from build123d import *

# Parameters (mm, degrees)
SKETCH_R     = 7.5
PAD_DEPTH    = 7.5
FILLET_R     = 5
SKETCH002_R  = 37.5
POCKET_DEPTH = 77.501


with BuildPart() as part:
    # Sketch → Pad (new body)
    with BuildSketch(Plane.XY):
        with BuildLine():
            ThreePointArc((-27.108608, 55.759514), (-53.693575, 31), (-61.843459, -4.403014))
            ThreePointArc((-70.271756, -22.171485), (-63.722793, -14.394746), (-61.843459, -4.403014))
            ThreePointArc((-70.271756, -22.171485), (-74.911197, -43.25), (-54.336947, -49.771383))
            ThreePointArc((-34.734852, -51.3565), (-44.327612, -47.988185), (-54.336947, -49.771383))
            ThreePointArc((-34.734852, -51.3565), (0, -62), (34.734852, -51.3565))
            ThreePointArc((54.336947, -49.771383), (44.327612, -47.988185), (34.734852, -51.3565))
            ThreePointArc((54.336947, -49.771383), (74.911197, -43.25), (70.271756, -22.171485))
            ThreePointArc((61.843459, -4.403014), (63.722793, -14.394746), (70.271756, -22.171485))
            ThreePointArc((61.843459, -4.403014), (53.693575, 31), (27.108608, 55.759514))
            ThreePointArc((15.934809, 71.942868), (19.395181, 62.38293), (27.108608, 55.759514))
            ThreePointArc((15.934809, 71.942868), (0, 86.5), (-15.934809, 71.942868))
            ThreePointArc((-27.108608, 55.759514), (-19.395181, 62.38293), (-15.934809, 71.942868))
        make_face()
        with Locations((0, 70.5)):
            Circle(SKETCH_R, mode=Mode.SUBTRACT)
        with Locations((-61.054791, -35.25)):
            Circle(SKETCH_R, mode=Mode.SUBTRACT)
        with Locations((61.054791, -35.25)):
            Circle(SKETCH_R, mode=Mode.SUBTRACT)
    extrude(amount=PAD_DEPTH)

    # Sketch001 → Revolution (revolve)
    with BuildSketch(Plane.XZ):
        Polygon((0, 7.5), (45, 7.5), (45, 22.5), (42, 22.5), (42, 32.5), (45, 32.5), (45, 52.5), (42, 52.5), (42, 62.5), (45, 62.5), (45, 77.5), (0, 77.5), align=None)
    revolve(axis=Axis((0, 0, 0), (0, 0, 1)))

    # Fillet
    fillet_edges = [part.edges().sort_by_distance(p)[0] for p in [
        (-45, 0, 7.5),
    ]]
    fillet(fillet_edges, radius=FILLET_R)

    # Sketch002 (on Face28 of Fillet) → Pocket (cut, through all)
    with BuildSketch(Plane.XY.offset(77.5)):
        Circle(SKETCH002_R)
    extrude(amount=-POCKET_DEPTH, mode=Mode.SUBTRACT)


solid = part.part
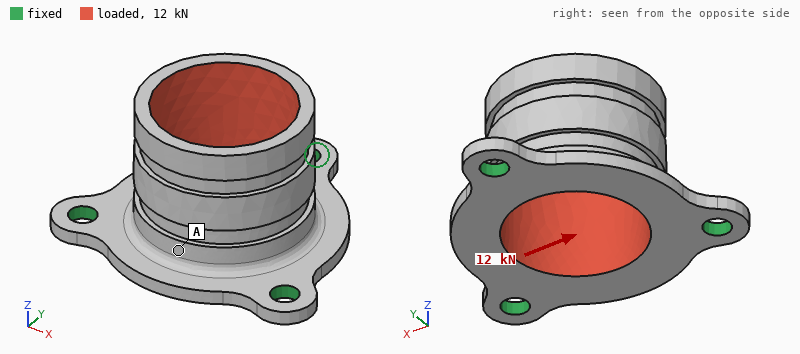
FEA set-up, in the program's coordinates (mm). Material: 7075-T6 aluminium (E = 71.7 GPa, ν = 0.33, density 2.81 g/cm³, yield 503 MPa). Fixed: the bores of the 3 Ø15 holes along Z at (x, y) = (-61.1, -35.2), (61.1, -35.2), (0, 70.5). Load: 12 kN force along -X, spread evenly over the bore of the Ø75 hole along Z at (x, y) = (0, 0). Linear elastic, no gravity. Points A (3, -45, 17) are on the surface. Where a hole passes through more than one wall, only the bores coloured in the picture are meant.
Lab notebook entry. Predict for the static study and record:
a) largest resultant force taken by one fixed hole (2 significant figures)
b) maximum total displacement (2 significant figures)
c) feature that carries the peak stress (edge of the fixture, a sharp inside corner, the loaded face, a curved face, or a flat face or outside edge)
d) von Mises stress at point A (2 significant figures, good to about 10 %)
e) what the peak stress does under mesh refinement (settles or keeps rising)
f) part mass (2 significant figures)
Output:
5.8 kN
0.21 mm
edge of the fixture
15 MPa
keeps rising
540 g
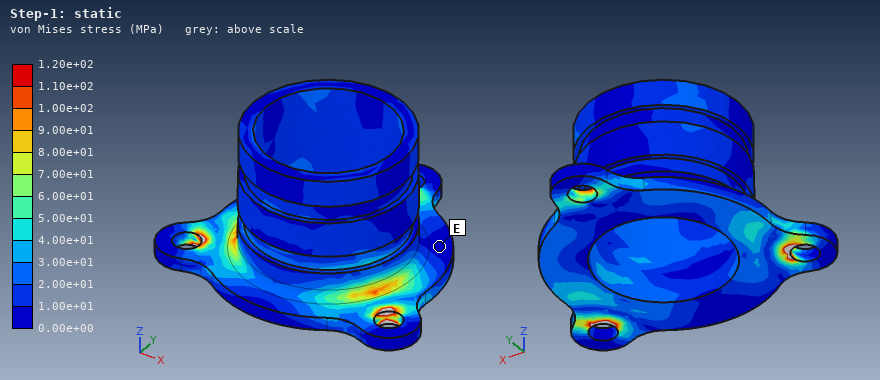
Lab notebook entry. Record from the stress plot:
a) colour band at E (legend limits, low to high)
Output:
0.00e+00 to 1.00e+01 MPa
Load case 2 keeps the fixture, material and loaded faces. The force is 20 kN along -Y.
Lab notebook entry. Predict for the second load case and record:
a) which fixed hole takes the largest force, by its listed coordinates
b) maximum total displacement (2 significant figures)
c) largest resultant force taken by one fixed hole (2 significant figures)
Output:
(0, 70.5)
0.37 mm
11 kN
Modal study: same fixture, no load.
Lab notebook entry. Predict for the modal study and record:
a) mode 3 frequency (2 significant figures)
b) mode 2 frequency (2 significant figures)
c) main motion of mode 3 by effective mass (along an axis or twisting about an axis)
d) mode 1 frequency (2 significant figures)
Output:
2900 Hz
2100 Hz
along Z
2100 Hz
